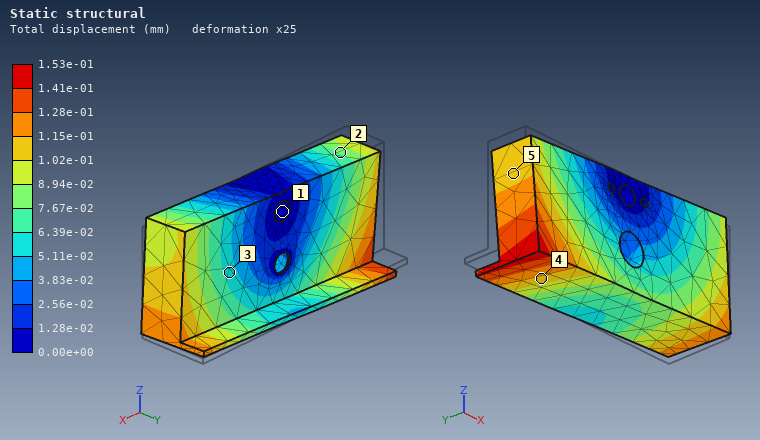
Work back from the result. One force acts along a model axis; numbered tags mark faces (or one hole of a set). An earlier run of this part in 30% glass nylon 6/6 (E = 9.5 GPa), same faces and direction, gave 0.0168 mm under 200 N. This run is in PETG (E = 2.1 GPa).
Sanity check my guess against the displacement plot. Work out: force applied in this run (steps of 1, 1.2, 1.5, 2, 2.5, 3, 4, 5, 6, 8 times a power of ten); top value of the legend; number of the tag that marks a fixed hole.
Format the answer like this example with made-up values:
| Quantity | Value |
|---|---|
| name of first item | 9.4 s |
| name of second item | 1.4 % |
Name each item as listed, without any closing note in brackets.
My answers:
| Quantity | Value |
|---|---|
| force applied in this run | 400 N |
| top value of the legend | 1.53e-01 mm |
| number of the tag that marks a fixed hole | 1 |
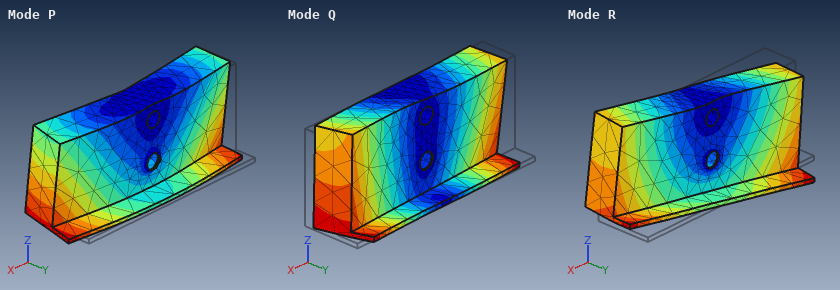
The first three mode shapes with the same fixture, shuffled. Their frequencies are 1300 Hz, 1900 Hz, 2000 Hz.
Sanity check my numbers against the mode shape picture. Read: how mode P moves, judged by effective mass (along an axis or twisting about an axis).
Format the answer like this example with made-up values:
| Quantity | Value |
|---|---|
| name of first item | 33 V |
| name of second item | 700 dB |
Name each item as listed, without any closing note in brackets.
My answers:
| Quantity | Value |
|---|---|
| how mode P moves, judged by effective mass | along Y |
